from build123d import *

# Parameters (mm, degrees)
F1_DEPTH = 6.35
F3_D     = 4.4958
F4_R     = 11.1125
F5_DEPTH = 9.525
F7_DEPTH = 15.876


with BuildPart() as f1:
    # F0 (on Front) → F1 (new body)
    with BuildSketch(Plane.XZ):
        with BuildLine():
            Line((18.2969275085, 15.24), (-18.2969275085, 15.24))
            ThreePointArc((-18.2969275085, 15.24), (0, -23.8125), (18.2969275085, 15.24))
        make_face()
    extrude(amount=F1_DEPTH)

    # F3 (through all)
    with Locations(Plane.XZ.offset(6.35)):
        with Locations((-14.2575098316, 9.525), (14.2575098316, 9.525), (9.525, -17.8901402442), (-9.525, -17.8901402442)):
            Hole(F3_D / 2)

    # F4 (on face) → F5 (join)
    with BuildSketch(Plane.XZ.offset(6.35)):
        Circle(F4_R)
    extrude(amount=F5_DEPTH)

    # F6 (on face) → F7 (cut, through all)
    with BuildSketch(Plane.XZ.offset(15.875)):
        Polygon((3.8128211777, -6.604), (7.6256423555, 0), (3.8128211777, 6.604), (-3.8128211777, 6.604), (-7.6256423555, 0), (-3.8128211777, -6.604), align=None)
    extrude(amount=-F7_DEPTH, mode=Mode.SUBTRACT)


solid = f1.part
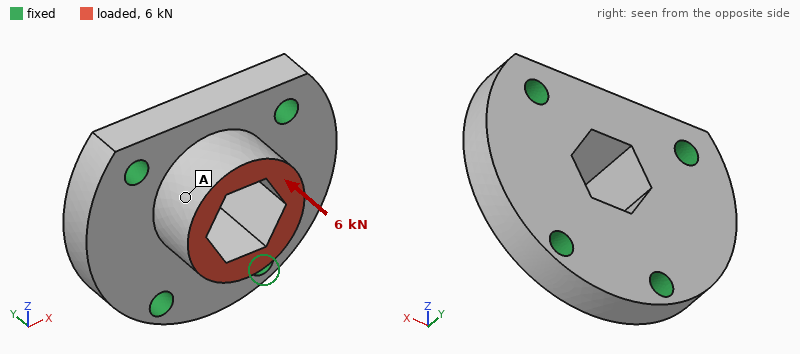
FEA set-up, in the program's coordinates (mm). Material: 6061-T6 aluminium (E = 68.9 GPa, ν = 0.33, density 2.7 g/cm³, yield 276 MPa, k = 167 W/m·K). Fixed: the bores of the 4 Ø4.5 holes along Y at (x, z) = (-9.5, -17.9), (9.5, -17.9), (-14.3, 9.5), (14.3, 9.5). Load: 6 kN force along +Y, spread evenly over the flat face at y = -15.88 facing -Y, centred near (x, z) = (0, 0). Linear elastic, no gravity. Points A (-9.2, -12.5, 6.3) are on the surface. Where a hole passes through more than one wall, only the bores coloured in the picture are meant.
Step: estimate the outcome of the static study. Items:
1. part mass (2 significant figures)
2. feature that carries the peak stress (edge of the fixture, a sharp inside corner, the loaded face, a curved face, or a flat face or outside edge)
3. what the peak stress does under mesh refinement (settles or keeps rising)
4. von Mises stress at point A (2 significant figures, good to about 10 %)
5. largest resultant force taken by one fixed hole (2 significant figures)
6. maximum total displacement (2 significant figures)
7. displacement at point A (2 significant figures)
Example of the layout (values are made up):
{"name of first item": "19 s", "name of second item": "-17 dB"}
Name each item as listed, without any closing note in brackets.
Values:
{"part mass": "29 g", "feature that carries the peak stress": "edge of the fixture", "what the peak stress does under mesh refinement": "keeps rising", "von Mises stress at point A": "26 MPa", "largest resultant force taken by one fixed hole": "2.0 kN", "maximum total displacement": "17 µm", "displacement at point A": "14 µm"}
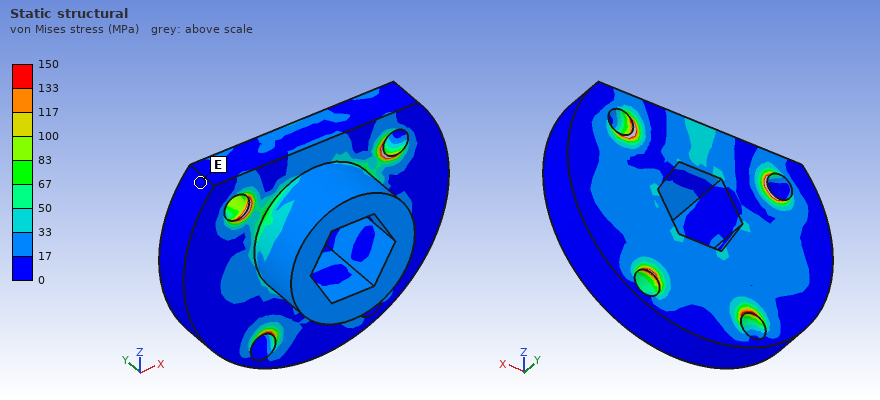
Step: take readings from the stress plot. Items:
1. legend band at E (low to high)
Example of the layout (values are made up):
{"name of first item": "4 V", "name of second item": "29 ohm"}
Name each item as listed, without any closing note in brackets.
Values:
{"legend band at E": "0 to 17 MPa"}
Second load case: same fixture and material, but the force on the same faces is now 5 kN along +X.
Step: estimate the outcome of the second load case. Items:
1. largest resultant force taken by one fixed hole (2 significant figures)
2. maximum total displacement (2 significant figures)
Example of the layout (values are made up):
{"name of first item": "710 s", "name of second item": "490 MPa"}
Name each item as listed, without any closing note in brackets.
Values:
{"largest resultant force taken by one fixed hole": "2.4 kN", "maximum total displacement": "43 µm"}
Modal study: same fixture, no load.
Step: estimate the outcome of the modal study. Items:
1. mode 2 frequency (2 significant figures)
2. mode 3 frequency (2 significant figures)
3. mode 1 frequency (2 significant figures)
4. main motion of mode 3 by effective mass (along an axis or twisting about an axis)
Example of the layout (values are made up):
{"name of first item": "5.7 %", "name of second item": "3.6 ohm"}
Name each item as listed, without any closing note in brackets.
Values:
{"mode 2 frequency": "27 kHz", "mode 3 frequency": "30 kHz", "mode 1 frequency": "27 kHz", "main motion of mode 3 by effective mass": "along Y"}
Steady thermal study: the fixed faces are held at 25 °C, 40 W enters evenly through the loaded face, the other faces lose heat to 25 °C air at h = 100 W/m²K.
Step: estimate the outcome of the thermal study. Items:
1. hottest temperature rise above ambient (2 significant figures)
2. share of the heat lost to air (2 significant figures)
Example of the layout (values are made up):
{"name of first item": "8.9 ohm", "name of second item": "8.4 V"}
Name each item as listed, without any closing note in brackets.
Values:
{"hottest temperature rise above ambient": "16 K", "share of the heat lost to air": "5.2 %"}
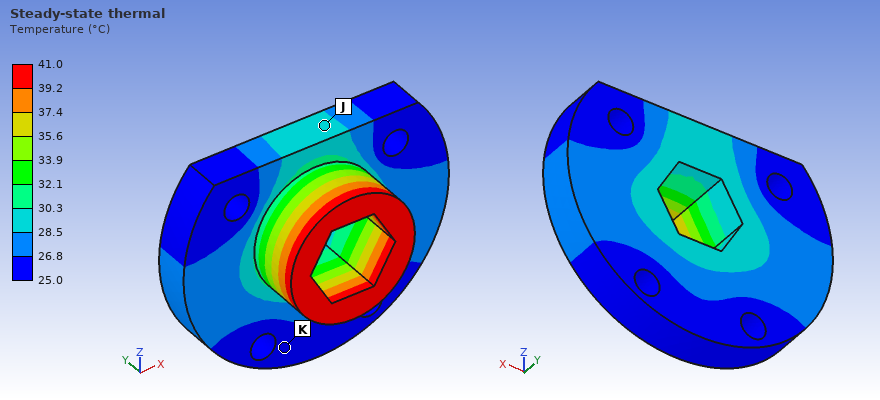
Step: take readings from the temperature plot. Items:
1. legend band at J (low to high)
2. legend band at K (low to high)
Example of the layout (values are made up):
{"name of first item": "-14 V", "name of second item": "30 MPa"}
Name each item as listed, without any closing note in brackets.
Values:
{"legend band at J": "28.5 to 30.3 °C", "legend band at K": "25.0 to 26.8 °C"}
